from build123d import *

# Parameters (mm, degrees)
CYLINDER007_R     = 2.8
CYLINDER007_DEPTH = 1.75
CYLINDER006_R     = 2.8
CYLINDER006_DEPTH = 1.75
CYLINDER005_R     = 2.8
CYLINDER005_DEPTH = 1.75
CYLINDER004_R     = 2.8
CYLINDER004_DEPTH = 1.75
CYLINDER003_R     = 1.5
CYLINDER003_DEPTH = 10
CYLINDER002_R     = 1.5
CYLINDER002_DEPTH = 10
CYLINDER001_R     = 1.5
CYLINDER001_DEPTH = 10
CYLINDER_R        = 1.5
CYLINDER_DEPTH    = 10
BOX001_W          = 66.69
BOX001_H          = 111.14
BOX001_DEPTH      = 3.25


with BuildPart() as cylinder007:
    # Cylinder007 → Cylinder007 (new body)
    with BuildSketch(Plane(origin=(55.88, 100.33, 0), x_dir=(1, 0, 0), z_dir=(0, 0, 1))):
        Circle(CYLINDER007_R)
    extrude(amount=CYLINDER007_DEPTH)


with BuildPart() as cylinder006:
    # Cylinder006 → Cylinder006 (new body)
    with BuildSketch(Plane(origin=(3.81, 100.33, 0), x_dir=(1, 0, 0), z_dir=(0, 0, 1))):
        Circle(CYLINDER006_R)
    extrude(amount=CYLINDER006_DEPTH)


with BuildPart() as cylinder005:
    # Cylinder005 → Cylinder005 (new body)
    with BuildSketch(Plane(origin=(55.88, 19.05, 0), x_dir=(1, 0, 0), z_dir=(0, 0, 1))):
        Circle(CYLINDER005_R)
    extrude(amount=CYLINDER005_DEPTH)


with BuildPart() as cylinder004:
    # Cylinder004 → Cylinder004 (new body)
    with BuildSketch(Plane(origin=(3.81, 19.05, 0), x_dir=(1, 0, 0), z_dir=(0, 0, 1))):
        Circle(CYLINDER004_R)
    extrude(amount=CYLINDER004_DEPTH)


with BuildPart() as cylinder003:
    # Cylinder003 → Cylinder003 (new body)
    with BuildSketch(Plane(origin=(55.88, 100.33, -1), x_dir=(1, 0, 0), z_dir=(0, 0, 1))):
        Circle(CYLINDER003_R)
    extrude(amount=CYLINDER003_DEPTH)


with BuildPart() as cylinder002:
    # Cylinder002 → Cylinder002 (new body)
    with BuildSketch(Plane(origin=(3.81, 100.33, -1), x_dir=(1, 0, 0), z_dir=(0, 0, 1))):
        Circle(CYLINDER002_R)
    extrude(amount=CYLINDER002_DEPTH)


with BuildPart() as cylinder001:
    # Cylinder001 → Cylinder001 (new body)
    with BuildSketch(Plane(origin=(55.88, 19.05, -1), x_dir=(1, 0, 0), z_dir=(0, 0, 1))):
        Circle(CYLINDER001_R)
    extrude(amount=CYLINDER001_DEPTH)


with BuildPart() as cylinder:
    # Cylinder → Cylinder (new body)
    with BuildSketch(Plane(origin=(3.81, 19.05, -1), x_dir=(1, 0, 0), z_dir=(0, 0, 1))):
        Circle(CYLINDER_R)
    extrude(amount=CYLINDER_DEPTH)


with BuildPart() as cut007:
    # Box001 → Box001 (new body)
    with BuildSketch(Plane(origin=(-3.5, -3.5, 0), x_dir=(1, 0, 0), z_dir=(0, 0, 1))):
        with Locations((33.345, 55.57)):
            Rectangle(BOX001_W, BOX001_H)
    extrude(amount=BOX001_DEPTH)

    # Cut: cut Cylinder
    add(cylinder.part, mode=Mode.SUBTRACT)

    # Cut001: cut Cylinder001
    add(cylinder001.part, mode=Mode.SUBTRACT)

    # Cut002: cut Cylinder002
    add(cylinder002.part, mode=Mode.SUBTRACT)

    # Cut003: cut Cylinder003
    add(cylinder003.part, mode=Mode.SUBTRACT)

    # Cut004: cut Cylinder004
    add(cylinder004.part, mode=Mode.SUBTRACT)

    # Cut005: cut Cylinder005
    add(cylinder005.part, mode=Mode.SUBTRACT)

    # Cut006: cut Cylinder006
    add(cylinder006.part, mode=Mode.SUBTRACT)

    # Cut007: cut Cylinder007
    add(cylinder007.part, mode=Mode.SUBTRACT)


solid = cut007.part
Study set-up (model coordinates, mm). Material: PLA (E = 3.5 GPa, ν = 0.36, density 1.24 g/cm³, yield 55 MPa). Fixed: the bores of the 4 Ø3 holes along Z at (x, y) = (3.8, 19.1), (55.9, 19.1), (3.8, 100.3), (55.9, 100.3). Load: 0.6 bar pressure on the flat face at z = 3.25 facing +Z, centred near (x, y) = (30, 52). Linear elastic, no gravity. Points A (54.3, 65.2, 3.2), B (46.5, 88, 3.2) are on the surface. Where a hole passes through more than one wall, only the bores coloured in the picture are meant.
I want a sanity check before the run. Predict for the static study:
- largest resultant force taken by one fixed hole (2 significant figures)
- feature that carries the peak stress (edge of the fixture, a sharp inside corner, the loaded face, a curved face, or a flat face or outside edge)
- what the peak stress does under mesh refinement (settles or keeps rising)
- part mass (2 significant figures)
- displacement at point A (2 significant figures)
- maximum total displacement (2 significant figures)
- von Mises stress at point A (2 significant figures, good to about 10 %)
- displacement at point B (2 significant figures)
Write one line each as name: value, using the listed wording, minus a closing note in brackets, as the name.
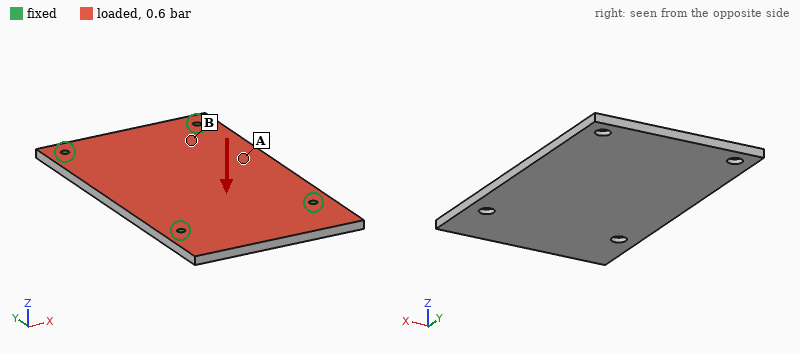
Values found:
largest resultant force taken by one fixed hole: 220 N
feature that carries the peak stress: edge of the fixture
what the peak stress does under mesh refinement: keeps rising
part mass: 30 g
displacement at point A: 1.2 mm
maximum total displacement: 1.3 mm
von Mises stress at point A: 11 MPa
displacement at point B: 0.58 mm
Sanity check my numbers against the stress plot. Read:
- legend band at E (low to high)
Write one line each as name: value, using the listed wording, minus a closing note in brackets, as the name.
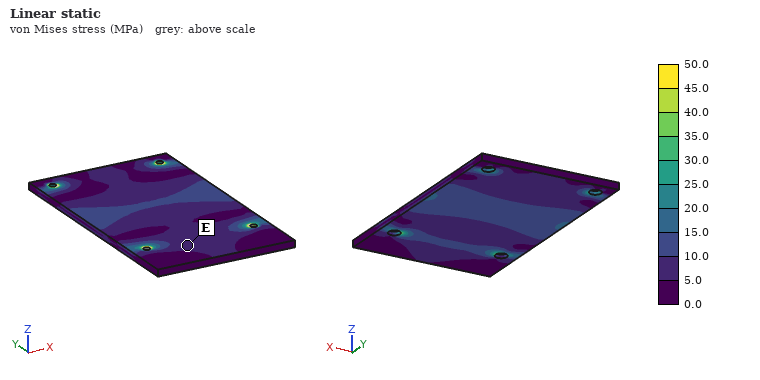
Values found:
legend band at E: 5.0 to 10.0 MPa
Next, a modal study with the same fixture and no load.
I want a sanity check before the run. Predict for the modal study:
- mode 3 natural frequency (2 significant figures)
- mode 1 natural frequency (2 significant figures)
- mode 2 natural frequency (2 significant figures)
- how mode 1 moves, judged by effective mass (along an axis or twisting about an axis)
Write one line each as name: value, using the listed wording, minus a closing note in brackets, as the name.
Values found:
mode 3 natural frequency: 970 Hz
mode 1 natural frequency: 580 Hz
mode 2 natural frequency: 930 Hz
how mode 1 moves, judged by effective mass: along Z
